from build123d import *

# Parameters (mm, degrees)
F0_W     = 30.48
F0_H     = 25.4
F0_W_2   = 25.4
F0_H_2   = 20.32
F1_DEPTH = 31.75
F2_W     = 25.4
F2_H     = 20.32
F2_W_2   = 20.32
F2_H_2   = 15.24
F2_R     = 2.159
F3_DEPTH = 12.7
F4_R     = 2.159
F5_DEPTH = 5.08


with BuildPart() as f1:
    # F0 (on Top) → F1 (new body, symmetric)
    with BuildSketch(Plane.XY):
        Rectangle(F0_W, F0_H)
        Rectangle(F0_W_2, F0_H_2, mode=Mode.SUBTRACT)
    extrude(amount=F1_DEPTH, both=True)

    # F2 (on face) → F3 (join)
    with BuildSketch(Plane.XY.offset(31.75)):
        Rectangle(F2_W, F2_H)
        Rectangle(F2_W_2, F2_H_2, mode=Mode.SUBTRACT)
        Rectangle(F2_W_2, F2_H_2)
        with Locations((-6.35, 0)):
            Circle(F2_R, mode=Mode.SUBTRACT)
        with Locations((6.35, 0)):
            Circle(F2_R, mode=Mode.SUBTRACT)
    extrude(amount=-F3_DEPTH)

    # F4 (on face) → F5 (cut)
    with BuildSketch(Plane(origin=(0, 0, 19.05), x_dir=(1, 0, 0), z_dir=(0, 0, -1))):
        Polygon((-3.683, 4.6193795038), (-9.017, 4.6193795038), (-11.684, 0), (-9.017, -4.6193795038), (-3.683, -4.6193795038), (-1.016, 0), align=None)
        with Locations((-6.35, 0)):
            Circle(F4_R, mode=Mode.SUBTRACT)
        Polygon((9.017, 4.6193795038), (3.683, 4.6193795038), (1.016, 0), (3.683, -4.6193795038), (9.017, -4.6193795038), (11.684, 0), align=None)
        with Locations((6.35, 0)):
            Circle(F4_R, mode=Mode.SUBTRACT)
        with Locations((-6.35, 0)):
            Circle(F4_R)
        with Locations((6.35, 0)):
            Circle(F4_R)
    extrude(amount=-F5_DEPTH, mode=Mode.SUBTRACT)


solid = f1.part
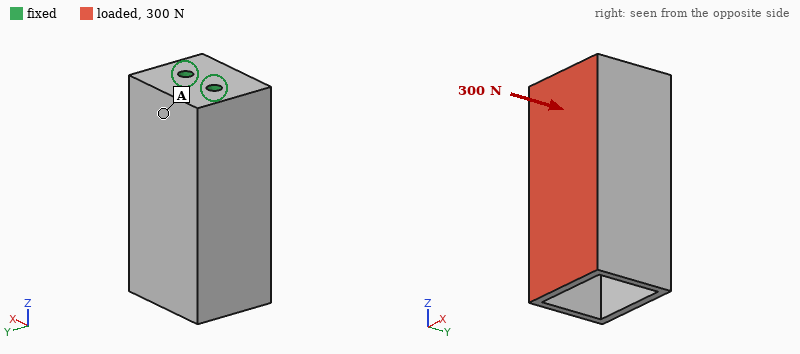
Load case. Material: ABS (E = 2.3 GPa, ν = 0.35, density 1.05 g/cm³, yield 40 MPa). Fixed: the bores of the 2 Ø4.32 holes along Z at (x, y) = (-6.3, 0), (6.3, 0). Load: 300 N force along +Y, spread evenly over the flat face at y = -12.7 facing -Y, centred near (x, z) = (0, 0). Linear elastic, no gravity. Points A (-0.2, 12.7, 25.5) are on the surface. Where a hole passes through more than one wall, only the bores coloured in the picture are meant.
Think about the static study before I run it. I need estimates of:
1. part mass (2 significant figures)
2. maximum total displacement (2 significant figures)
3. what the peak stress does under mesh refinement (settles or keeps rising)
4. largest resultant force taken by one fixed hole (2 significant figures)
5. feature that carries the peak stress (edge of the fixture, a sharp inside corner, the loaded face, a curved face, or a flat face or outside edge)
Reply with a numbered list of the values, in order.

1. 23 g
2. 0.89 mm
3. keeps rising
4. 150 N
5. edge of the fixture
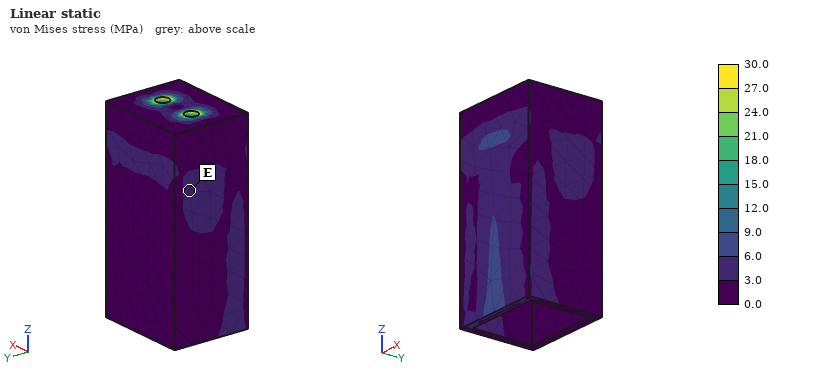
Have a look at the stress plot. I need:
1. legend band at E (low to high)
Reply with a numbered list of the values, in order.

1. 3.0 to 6.0 MPa
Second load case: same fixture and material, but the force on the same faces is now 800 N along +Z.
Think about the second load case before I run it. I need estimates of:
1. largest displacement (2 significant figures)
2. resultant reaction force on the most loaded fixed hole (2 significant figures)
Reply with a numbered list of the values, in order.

1. 0.90 mm
2. 400 N
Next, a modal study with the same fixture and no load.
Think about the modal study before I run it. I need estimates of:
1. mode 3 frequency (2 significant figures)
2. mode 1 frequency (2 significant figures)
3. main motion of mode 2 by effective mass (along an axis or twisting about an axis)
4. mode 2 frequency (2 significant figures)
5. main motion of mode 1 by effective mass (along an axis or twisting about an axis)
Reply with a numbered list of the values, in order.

1. 1900 Hz
2. 930 Hz
3. along X
4. 1300 Hz
5. along Y
